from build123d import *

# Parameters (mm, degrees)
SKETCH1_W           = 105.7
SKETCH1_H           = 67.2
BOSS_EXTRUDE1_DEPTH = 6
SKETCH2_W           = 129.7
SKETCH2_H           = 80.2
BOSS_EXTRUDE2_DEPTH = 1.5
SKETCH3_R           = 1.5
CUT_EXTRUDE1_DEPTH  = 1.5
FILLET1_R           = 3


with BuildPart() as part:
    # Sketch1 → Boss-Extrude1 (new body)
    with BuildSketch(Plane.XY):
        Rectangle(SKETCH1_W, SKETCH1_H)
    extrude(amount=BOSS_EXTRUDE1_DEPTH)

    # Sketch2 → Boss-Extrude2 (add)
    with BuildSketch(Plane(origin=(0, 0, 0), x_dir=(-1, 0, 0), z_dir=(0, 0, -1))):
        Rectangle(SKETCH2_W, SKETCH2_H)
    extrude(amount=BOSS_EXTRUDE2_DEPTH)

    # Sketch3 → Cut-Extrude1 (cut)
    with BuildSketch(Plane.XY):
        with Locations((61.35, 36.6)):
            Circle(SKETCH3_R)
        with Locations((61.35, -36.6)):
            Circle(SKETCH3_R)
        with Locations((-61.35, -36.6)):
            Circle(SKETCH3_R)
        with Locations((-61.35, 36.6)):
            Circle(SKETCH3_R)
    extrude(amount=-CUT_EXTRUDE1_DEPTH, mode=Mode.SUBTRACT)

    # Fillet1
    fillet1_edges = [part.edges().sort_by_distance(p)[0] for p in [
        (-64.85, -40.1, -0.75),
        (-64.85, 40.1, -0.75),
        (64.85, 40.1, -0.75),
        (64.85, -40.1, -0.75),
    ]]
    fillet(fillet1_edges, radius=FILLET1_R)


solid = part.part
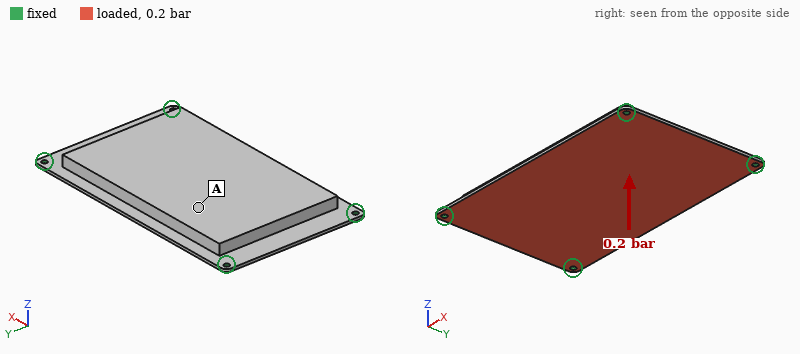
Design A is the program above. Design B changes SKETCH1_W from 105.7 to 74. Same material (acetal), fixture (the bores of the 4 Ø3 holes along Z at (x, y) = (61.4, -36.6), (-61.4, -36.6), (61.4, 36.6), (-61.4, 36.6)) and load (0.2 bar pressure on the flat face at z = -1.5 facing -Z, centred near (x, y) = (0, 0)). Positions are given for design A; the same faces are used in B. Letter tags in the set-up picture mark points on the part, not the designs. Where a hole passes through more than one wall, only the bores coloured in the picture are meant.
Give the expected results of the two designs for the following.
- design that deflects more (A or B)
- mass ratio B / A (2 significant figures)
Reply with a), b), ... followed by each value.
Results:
a) B
b) 0.78
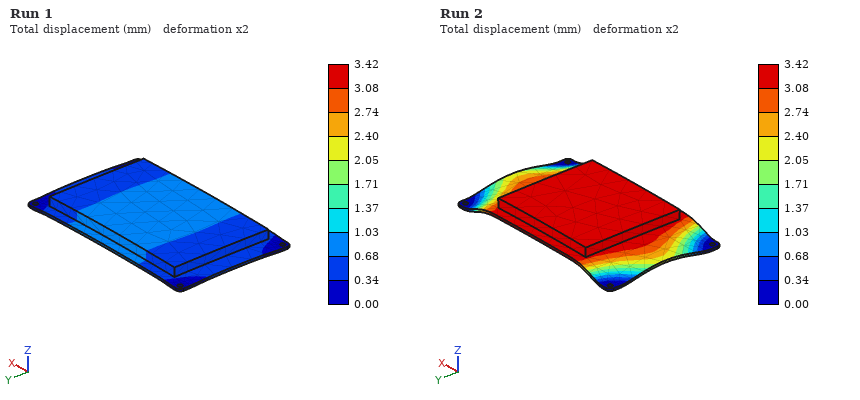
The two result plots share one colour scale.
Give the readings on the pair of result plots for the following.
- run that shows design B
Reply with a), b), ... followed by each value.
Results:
a) Run 2
